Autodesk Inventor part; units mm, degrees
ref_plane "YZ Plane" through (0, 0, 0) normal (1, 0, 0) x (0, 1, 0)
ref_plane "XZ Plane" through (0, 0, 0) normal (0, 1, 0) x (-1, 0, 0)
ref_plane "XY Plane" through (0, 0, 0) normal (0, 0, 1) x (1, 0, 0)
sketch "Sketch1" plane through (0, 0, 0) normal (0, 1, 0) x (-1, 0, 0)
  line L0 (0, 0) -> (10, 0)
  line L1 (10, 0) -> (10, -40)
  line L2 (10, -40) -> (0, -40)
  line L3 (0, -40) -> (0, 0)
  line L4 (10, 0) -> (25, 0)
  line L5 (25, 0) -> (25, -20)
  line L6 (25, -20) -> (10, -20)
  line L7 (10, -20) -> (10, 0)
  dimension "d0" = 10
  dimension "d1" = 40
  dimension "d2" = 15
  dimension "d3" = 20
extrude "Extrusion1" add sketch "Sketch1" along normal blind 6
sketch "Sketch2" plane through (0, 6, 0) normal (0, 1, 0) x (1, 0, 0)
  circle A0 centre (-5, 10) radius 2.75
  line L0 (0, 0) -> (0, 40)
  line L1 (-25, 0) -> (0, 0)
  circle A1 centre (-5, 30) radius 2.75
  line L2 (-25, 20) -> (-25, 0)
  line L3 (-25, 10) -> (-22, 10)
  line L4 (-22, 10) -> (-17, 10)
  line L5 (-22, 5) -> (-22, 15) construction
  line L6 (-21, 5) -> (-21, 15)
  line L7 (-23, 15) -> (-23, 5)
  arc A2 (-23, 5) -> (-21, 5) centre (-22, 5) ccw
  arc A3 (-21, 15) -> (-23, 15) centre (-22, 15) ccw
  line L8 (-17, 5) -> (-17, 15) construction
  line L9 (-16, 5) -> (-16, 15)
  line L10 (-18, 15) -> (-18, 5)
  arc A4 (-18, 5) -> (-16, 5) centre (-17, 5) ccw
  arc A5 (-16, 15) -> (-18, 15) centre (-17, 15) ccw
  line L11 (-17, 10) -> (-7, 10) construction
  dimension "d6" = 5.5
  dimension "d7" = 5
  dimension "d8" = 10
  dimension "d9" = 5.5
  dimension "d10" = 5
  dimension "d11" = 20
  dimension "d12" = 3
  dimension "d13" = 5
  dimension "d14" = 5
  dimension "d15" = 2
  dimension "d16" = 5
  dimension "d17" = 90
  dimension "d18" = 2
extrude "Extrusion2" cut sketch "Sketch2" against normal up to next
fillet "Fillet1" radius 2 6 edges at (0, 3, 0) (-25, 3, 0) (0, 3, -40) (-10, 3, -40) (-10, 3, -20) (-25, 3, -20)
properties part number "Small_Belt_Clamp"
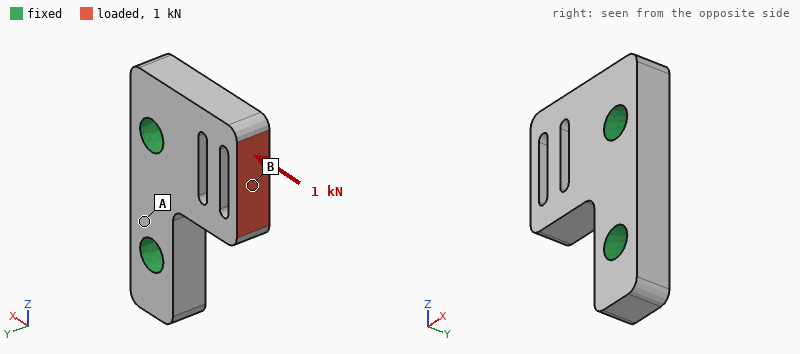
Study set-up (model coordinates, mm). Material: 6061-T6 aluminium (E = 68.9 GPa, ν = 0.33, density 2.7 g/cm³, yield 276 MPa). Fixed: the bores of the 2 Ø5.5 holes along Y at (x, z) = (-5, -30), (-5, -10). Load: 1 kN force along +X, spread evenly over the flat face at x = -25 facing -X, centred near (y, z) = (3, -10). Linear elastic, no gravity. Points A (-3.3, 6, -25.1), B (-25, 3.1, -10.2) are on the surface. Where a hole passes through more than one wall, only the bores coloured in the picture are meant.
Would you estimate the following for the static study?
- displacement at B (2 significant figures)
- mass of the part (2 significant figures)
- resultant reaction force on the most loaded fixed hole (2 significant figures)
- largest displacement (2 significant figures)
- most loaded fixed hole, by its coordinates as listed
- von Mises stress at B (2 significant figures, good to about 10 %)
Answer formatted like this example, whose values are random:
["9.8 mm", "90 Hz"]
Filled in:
["30 µm", "9.8 g", "910 N", "32 µm", "(-5, -10)", "130 MPa"]
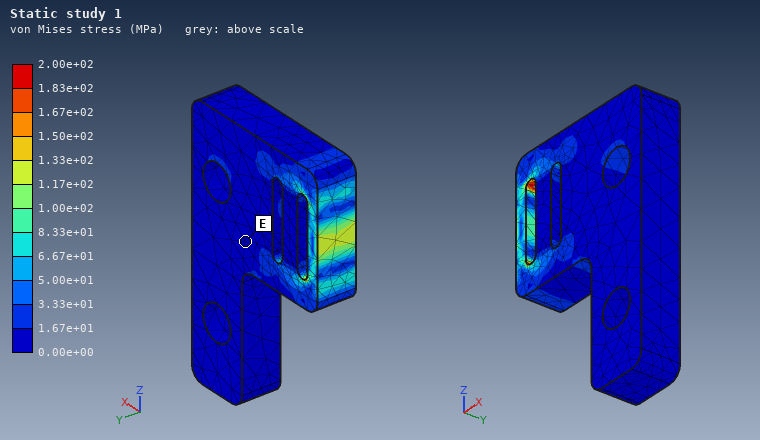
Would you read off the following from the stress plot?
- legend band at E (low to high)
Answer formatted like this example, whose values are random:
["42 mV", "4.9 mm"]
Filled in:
["0.00e+00 to 1.67e+01 MPa"]
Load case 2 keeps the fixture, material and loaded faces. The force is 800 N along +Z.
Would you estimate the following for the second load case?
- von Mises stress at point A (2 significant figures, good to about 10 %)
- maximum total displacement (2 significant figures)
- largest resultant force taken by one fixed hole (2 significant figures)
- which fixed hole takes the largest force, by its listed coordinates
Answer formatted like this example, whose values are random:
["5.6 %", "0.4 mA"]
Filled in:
["18 MPa", "43 µm", "700 N", "(-5, -10)"]
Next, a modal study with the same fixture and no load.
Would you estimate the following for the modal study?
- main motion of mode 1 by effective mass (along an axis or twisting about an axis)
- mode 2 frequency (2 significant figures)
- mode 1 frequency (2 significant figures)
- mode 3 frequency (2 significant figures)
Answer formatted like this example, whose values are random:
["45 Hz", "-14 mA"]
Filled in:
["along Y", "20 kHz", "12 kHz", "20 kHz"]
